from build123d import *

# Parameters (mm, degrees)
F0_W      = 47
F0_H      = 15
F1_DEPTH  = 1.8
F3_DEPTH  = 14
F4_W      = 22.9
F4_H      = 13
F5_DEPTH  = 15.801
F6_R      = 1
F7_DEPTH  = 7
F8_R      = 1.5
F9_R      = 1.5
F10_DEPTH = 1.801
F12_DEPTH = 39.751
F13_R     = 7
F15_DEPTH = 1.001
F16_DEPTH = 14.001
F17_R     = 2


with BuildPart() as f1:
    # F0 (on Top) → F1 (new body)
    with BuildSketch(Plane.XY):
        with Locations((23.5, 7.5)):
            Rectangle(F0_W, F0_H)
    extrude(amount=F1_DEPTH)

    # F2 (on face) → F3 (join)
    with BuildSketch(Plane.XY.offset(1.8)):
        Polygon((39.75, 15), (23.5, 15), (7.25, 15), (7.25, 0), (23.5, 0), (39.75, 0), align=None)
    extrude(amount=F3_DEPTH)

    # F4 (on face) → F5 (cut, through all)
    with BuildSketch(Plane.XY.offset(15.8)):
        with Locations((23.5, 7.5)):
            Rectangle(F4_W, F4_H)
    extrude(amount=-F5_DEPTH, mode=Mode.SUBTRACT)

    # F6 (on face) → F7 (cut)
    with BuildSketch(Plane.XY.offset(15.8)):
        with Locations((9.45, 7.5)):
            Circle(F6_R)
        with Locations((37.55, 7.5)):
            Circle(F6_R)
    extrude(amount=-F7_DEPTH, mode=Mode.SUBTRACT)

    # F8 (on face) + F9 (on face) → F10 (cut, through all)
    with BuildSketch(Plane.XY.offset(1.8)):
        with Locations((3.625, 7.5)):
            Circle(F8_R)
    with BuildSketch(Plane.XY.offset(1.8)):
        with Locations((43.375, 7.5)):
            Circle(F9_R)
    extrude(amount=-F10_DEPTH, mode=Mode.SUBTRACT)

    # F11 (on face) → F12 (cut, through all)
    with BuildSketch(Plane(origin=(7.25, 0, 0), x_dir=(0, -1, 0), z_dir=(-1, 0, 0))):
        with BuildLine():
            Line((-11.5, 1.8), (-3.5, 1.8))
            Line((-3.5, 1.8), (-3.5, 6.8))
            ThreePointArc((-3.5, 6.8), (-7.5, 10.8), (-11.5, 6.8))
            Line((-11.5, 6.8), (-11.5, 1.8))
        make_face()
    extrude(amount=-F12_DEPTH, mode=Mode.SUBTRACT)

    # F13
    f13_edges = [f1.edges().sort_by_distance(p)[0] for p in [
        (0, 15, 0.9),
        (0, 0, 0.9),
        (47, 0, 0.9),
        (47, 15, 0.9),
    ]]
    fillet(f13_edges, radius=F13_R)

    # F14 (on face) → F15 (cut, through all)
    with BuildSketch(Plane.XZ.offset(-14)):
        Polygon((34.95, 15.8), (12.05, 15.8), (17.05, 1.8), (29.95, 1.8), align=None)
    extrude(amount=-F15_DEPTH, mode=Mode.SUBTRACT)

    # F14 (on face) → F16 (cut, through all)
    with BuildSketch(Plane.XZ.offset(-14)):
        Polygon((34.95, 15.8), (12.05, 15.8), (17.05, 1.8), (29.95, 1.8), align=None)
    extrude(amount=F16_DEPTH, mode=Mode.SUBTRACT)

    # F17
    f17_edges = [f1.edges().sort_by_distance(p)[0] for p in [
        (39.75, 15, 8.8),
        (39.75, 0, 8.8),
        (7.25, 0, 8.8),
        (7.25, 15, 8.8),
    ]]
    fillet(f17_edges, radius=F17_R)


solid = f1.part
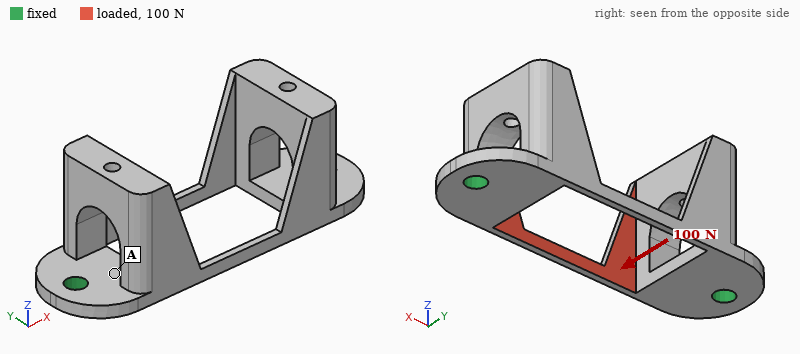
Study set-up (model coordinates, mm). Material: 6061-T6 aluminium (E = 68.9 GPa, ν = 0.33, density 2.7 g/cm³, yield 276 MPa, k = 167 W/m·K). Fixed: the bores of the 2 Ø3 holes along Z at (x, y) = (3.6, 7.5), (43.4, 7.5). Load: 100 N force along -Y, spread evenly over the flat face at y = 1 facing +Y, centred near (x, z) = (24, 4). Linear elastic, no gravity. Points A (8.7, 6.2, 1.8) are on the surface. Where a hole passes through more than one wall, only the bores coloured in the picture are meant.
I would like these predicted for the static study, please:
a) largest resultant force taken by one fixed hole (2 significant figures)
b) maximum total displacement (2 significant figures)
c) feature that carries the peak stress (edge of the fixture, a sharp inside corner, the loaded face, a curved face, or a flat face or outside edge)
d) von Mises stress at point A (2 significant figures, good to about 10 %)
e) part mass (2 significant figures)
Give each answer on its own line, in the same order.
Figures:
51 N
86 µm
a flat face or outside edge
11 MPa
5.6 g
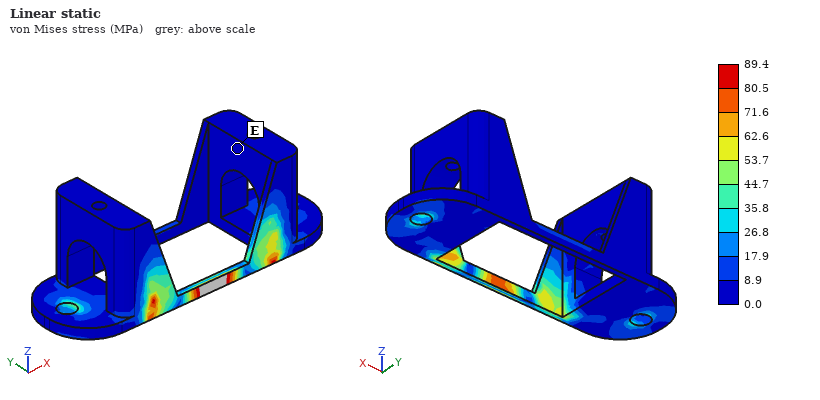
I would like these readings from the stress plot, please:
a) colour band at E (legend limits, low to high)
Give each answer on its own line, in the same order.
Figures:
0.0 to 8.9 MPa
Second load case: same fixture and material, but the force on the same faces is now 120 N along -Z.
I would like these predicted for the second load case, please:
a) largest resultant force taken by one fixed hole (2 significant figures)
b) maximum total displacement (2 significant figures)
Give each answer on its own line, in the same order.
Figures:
61 N
97 µm
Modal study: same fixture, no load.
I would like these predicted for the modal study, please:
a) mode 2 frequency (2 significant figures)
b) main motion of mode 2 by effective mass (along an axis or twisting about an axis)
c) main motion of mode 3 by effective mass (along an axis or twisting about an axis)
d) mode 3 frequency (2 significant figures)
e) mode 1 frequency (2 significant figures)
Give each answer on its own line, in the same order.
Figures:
4400 Hz
along Y
twisting about Z
4700 Hz
3300 Hz
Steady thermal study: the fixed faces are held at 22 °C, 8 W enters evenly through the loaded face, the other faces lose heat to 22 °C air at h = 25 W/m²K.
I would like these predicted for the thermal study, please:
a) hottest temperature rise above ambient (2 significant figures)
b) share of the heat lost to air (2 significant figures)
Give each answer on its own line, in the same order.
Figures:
32 K
5.4 %
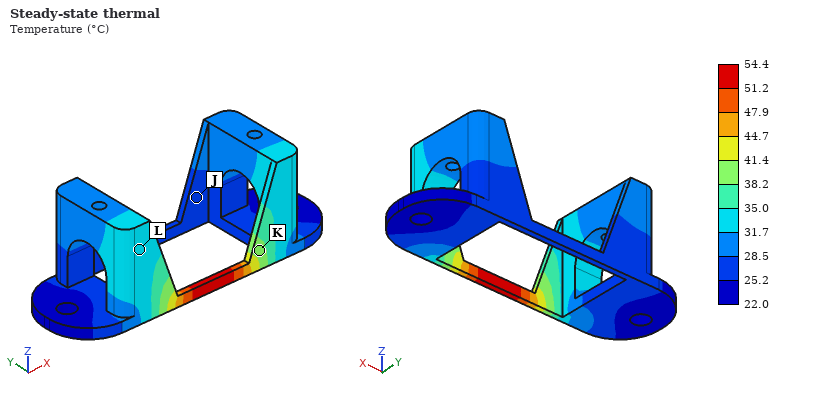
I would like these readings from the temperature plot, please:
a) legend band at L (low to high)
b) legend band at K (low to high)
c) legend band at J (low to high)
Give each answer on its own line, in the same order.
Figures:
31.7 to 35.0 °C
38.2 to 41.4 °C
25.2 to 28.5 °C
